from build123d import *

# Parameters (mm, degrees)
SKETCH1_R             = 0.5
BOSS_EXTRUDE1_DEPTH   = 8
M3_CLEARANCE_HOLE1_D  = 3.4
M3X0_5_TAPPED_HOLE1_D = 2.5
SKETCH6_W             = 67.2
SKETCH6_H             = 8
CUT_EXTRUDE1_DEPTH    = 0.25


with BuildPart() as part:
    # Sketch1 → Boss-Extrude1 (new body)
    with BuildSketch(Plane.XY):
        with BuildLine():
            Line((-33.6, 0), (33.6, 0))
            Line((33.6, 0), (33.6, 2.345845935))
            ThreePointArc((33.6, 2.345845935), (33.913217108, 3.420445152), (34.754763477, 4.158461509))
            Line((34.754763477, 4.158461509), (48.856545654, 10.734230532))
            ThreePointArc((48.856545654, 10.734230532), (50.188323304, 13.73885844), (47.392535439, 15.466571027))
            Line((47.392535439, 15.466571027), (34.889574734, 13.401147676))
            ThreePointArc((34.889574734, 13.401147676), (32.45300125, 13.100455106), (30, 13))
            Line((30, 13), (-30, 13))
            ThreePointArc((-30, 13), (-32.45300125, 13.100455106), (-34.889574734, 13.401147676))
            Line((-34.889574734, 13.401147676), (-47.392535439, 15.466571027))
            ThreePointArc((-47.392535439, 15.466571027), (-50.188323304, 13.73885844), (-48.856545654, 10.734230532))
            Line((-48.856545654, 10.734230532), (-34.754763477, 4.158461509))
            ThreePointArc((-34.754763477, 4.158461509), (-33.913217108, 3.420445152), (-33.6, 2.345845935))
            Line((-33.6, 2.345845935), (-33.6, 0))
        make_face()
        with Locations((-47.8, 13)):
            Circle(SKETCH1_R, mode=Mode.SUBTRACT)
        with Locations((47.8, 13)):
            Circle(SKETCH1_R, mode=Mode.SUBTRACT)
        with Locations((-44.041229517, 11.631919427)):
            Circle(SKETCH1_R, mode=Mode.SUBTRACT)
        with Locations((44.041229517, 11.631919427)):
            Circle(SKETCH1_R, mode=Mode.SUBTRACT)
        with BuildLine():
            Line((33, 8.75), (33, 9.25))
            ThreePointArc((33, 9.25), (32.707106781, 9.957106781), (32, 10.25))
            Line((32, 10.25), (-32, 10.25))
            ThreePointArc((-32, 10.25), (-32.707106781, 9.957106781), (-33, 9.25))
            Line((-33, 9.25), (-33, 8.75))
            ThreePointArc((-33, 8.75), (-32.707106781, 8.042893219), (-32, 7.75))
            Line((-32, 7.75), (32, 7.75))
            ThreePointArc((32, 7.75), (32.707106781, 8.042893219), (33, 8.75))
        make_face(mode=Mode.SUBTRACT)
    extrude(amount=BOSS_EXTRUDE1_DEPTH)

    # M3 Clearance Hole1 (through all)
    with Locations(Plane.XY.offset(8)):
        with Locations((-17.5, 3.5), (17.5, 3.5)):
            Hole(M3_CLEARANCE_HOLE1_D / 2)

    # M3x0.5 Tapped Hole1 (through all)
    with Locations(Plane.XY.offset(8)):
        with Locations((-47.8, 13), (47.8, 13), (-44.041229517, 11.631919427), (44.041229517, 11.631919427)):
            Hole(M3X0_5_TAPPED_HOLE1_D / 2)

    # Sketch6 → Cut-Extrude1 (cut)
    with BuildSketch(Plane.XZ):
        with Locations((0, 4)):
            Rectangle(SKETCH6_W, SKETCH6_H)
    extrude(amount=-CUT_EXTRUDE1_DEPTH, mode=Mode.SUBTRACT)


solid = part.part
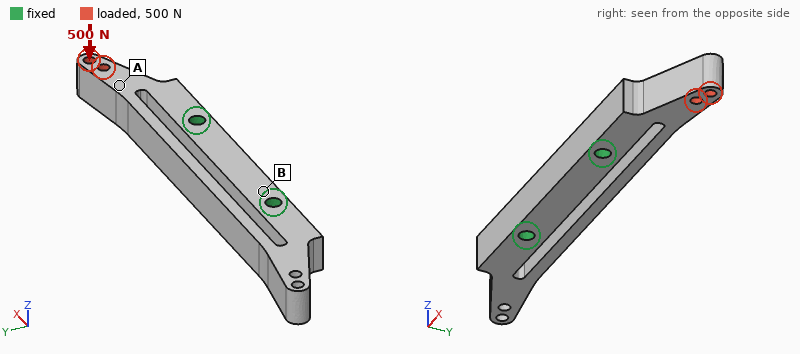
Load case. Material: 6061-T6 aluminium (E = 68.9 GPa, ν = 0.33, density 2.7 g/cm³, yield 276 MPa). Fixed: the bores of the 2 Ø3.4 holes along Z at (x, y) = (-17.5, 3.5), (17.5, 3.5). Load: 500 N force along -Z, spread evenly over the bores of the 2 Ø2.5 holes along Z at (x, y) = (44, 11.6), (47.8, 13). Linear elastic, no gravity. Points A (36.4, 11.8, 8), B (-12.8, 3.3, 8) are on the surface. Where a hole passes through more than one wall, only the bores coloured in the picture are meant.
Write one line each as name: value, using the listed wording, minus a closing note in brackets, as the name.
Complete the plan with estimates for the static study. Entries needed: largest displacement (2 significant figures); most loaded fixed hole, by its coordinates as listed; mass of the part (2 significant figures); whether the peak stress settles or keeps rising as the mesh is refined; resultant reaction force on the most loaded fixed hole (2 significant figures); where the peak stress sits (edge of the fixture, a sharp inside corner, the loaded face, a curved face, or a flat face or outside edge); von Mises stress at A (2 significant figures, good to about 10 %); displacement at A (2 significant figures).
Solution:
largest displacement: 0.25 mm
most loaded fixed hole, by its coordinates as listed: (17.5, 3.5)
mass of the part: 19 g
whether the peak stress settles or keeps rising as the mesh is refined: keeps rising
resultant reaction force on the most loaded fixed hole: 550 N
where the peak stress sits: edge of the fixture
von Mises stress at A: 50 MPa
displacement at A: 0.12 mm
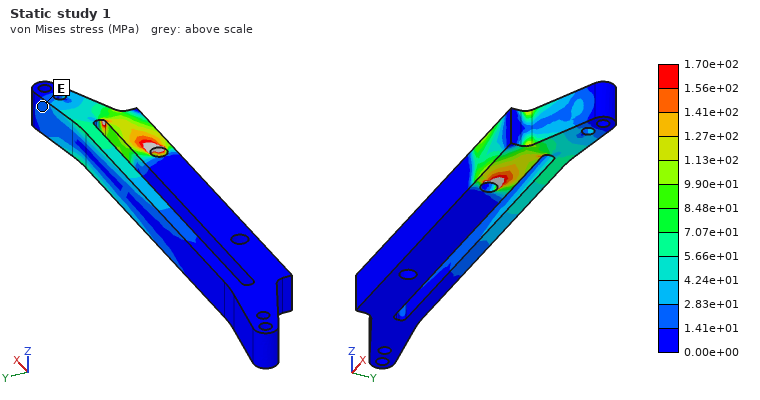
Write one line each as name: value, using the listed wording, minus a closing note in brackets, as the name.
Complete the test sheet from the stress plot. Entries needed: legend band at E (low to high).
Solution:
legend band at E: 1.41e+01 to 2.83e+01 MPa
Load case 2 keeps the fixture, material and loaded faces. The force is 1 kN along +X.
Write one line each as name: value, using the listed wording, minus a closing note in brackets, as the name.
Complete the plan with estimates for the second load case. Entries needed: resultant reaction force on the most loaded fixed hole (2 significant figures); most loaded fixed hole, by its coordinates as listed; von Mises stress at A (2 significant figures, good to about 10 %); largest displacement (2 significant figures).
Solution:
resultant reaction force on the most loaded fixed hole: 560 N
most loaded fixed hole, by its coordinates as listed: (17.5, 3.5)
von Mises stress at A: 29 MPa
largest displacement: 0.18 mm
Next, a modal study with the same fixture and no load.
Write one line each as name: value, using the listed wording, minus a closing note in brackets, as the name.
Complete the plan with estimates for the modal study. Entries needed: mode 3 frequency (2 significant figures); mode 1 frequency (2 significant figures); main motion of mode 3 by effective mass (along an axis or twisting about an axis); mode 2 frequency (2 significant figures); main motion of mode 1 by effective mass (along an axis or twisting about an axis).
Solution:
mode 3 frequency: 5500 Hz
mode 1 frequency: 3000 Hz
main motion of mode 3 by effective mass: along Z
mode 2 frequency: 5100 Hz
main motion of mode 1 by effective mass: along Y
